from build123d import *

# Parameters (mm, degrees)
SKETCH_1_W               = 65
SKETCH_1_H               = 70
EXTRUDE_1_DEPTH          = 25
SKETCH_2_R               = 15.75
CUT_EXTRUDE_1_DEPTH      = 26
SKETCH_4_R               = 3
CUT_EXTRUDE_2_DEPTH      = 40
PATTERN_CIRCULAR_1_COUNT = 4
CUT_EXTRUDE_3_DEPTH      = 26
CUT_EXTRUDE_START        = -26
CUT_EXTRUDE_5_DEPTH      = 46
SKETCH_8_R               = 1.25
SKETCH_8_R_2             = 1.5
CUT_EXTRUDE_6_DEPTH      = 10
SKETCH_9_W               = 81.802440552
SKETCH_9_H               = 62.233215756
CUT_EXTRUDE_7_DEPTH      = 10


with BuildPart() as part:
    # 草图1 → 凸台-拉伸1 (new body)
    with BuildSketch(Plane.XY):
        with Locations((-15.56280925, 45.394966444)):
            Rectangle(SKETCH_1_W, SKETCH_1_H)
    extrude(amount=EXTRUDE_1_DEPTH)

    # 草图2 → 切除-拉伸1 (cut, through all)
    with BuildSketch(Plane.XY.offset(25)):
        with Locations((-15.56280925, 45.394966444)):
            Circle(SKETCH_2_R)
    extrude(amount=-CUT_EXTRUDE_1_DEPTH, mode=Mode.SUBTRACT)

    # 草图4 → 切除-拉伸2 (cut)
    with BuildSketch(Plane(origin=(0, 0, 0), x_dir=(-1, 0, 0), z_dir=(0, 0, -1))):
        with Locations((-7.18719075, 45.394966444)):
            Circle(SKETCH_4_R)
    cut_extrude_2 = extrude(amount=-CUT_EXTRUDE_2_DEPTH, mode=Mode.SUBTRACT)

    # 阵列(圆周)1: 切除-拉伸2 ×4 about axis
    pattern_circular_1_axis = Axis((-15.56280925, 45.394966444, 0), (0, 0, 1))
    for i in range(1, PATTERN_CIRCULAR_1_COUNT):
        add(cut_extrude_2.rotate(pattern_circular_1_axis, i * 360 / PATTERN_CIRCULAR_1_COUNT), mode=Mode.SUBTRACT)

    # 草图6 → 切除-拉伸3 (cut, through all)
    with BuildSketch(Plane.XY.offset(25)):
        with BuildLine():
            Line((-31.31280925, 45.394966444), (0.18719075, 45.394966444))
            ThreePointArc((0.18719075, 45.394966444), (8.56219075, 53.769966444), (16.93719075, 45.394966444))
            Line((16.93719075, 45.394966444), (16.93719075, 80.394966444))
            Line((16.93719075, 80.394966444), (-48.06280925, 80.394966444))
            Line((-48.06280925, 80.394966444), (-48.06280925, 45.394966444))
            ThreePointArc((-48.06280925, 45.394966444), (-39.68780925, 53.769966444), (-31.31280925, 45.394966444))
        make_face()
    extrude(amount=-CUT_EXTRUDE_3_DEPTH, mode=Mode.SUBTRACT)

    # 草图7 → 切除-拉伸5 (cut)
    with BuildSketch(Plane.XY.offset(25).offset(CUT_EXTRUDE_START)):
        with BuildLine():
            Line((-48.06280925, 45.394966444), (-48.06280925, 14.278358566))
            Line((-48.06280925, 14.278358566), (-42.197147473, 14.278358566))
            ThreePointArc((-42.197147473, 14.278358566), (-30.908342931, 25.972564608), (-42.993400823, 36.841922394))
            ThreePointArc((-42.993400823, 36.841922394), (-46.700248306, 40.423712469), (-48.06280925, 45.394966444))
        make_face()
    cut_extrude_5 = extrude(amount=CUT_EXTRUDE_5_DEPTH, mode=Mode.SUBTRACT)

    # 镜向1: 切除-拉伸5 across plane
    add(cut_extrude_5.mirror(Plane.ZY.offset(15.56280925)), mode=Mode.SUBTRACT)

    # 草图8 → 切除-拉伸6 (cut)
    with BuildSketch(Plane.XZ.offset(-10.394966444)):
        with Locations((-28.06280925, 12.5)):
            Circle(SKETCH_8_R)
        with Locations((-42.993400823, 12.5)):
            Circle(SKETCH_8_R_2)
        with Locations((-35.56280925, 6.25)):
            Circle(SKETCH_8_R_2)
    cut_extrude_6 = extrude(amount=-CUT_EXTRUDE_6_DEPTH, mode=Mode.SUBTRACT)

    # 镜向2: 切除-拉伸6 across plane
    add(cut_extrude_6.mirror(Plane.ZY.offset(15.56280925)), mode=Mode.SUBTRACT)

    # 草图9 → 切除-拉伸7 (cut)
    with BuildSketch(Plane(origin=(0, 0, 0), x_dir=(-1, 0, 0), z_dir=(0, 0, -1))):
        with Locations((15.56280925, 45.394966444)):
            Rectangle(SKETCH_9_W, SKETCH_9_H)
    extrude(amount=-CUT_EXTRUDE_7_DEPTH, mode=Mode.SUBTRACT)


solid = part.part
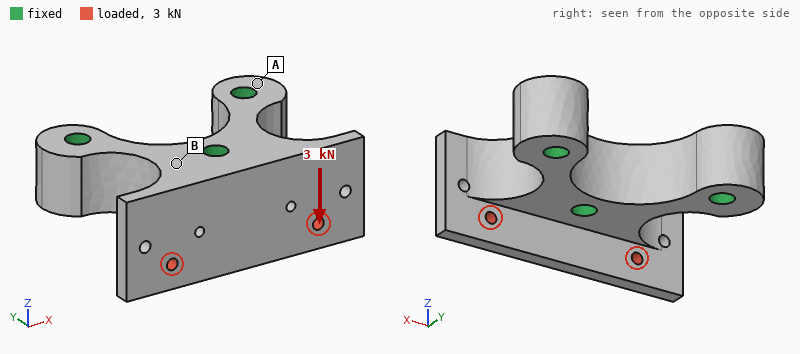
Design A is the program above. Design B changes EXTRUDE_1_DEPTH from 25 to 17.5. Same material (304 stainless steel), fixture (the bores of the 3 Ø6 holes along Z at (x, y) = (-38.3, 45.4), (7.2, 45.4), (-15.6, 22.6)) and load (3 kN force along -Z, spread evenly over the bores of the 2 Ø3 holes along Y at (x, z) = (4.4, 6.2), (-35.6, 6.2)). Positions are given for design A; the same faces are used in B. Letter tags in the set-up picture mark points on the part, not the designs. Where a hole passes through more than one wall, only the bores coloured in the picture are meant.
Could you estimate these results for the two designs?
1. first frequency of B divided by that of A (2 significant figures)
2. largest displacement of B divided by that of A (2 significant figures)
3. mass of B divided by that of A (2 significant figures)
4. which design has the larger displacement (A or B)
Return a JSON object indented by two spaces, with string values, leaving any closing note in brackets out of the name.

{
  "first frequency of B divided by that of A": "0.65",
  "largest displacement of B divided by that of A": "3.2",
  "mass of B divided by that of A": "0.55",
  "which design has the larger displacement": "B"
}
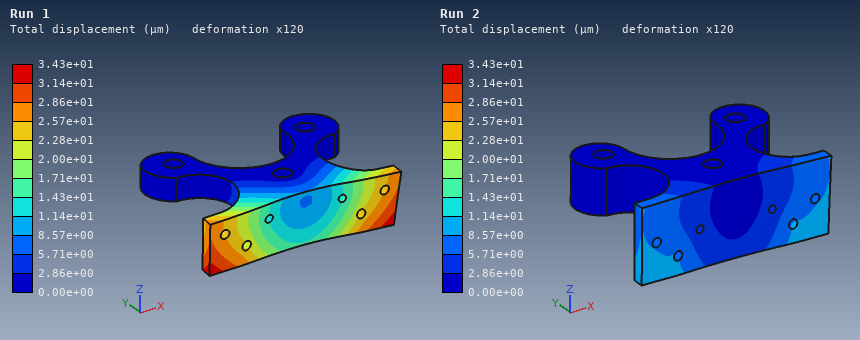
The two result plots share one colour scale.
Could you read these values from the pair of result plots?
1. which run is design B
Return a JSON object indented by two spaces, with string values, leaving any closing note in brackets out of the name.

{
  "which run is design B": "Run 1"
}
